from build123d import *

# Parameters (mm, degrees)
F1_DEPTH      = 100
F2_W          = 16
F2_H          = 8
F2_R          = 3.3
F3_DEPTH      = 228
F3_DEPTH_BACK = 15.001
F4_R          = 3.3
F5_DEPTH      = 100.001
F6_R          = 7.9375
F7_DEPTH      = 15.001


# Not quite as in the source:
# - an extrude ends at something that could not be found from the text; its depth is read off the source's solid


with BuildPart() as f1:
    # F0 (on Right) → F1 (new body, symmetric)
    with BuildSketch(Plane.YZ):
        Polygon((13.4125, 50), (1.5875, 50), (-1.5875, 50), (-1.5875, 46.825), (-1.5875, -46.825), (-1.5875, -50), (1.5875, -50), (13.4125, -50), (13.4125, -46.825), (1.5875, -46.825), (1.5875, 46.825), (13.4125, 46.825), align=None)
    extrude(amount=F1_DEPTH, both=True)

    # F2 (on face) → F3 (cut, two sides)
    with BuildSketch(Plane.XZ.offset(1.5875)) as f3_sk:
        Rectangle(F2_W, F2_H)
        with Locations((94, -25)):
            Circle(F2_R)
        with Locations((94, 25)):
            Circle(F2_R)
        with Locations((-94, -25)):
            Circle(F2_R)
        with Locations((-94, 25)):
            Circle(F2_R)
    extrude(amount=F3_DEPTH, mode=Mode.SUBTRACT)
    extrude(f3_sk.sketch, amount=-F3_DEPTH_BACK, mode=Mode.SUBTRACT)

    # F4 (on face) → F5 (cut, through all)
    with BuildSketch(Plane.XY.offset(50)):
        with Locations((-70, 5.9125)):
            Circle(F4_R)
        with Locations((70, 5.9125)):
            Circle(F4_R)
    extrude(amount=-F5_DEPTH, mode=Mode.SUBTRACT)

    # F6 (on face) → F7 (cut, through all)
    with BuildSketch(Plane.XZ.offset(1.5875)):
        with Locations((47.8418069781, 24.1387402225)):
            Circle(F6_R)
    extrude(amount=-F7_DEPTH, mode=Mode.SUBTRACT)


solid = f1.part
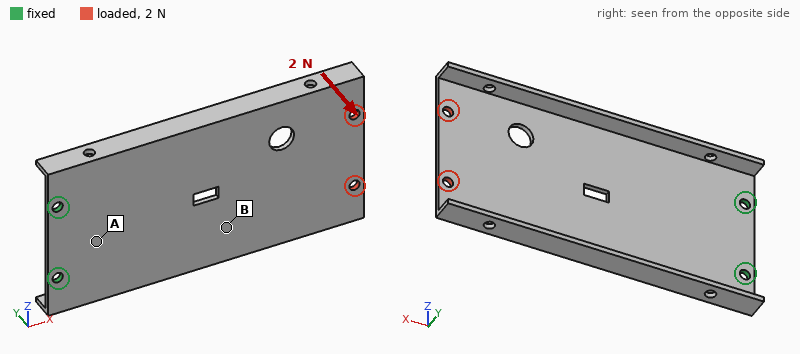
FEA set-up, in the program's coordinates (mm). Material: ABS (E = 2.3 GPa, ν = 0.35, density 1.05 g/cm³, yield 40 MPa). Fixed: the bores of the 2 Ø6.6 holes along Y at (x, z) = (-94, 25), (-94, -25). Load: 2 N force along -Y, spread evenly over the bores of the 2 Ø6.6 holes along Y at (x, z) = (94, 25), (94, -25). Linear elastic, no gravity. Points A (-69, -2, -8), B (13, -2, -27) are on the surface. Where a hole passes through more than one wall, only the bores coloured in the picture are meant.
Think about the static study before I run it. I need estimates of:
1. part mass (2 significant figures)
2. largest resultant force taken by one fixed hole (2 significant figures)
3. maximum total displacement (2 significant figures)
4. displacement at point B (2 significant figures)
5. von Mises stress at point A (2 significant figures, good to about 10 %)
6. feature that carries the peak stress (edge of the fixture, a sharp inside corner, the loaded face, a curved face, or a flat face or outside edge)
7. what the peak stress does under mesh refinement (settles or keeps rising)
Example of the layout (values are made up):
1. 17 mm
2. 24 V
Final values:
1. 80 g
2. 5.7 N
3. 2.3 mm
4. 1.1 mm
5. 0.76 MPa
6. edge of the fixture
7. keeps rising
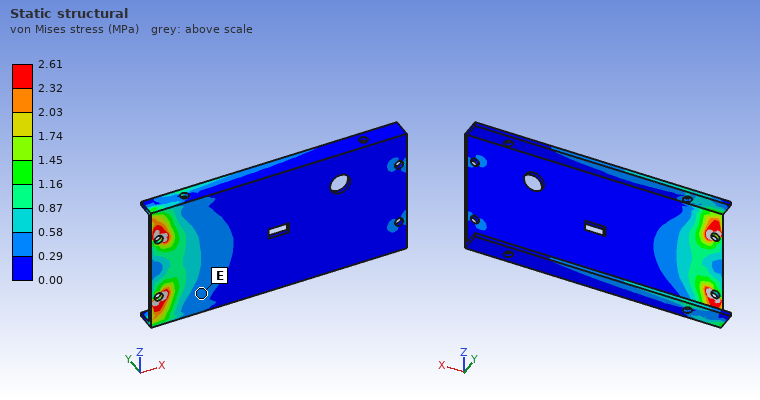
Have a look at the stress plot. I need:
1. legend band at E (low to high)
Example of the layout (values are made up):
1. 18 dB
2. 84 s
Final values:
1. 0.29 to 0.58 MPa
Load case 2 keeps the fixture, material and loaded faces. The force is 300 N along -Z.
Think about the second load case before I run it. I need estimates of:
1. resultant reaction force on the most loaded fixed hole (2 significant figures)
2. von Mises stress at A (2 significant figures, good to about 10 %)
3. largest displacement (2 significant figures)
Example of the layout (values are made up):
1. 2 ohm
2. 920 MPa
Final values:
1. 1.0 kN
2. 7.5 MPa
3. 2.3 mm
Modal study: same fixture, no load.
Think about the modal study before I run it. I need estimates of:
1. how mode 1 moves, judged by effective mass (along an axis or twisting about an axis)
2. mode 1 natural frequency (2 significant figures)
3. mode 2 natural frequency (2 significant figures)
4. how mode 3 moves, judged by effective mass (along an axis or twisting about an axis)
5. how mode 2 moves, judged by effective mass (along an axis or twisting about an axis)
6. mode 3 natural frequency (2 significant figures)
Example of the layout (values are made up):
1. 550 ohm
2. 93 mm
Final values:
1. along Y
2. 30 Hz
3. 74 Hz
4. along Y
5. twisting about X
6. 280 Hz
